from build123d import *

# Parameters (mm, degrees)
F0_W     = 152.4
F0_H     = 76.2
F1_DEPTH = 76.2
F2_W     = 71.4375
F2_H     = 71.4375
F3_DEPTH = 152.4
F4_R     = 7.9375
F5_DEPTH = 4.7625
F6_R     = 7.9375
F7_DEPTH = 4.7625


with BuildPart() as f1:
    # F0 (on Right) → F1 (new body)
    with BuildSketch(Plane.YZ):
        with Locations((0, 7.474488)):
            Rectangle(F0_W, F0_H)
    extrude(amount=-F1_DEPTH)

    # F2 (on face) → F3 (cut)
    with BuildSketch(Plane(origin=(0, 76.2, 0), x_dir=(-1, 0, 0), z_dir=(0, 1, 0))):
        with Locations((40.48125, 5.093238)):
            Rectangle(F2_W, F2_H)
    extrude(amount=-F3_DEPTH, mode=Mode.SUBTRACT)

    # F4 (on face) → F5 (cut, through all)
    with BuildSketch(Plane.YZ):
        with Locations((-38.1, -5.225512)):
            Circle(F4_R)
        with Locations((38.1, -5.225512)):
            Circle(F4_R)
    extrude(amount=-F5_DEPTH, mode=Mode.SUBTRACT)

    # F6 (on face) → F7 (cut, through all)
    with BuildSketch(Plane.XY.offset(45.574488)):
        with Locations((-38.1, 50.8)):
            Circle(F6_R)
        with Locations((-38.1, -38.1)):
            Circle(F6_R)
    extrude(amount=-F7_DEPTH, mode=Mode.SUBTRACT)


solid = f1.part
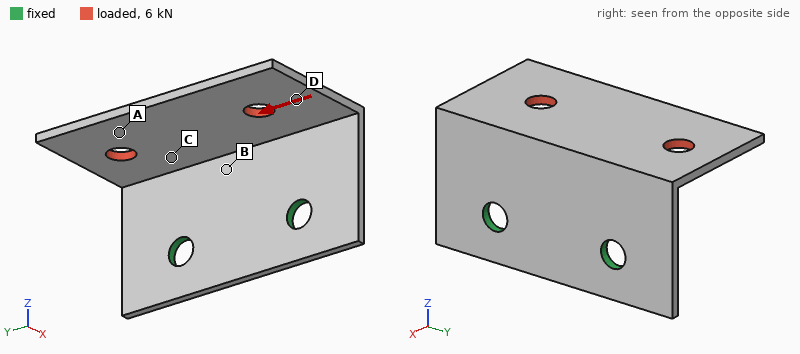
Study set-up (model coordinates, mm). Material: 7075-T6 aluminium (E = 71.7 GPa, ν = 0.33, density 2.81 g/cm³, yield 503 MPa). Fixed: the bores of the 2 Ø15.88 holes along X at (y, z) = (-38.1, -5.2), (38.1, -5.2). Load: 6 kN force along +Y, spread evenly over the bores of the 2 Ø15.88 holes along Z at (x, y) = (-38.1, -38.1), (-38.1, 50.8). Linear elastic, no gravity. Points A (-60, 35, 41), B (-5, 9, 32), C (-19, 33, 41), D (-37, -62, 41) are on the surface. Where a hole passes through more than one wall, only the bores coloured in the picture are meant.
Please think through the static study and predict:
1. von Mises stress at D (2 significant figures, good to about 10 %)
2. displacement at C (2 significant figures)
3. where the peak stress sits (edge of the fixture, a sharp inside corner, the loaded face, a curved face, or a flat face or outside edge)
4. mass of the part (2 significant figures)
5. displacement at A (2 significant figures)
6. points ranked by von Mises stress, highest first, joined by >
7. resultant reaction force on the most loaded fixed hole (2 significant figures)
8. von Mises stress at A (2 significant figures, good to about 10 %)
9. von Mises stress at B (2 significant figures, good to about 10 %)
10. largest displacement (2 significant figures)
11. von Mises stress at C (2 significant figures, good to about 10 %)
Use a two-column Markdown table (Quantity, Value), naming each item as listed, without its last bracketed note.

| Quantity | Value |
|---|---|
| von Mises stress at D | 58 MPa |
| displacement at C | 0.70 mm |
| where the peak stress sits | a flat face or outside edge |
| mass of the part | 290 g |
| displacement at A | 1.3 mm |
| points ranked by von Mises stress, highest first, joined by > | B > C > D > A |
| resultant reaction force on the most loaded fixed hole | 4.9 kN |
| von Mises stress at A | 27 MPa |
| von Mises stress at B | 140 MPa |
| largest displacement | 2.2 mm |
| von Mises stress at C | 95 MPa |
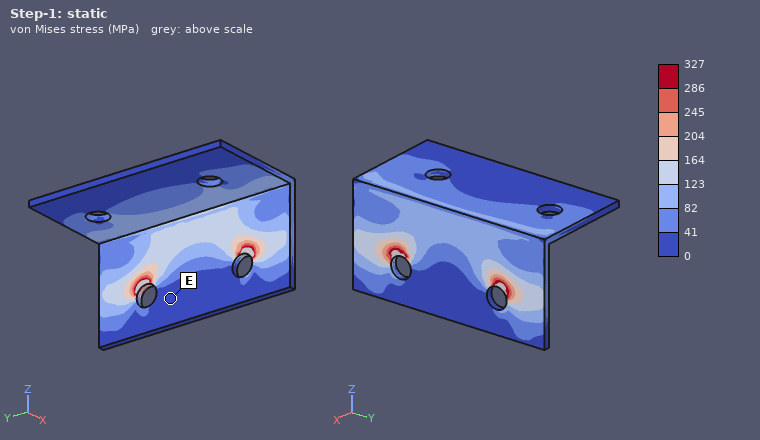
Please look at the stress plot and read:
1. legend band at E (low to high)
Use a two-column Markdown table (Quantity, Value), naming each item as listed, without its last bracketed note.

| Quantity | Value |
|---|---|
| legend band at E | 0 to 41 MPa |
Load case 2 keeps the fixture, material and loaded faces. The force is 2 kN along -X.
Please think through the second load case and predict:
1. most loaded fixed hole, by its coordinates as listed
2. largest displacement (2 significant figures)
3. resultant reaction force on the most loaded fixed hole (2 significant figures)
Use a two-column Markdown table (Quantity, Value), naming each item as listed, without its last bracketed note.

| Quantity | Value |
|---|---|
| most loaded fixed hole, by its coordinates as listed | (38.1, -5.2) |
| largest displacement | 1.7 mm |
| resultant reaction force on the most loaded fixed hole | 1.1 kN |
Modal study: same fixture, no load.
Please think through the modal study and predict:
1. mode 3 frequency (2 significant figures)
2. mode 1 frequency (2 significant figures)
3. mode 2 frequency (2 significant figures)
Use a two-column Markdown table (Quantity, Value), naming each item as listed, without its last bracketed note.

| Quantity | Value |
|---|---|
| mode 3 frequency | 1000 Hz |
| mode 1 frequency | 370 Hz |
| mode 2 frequency | 630 Hz |
